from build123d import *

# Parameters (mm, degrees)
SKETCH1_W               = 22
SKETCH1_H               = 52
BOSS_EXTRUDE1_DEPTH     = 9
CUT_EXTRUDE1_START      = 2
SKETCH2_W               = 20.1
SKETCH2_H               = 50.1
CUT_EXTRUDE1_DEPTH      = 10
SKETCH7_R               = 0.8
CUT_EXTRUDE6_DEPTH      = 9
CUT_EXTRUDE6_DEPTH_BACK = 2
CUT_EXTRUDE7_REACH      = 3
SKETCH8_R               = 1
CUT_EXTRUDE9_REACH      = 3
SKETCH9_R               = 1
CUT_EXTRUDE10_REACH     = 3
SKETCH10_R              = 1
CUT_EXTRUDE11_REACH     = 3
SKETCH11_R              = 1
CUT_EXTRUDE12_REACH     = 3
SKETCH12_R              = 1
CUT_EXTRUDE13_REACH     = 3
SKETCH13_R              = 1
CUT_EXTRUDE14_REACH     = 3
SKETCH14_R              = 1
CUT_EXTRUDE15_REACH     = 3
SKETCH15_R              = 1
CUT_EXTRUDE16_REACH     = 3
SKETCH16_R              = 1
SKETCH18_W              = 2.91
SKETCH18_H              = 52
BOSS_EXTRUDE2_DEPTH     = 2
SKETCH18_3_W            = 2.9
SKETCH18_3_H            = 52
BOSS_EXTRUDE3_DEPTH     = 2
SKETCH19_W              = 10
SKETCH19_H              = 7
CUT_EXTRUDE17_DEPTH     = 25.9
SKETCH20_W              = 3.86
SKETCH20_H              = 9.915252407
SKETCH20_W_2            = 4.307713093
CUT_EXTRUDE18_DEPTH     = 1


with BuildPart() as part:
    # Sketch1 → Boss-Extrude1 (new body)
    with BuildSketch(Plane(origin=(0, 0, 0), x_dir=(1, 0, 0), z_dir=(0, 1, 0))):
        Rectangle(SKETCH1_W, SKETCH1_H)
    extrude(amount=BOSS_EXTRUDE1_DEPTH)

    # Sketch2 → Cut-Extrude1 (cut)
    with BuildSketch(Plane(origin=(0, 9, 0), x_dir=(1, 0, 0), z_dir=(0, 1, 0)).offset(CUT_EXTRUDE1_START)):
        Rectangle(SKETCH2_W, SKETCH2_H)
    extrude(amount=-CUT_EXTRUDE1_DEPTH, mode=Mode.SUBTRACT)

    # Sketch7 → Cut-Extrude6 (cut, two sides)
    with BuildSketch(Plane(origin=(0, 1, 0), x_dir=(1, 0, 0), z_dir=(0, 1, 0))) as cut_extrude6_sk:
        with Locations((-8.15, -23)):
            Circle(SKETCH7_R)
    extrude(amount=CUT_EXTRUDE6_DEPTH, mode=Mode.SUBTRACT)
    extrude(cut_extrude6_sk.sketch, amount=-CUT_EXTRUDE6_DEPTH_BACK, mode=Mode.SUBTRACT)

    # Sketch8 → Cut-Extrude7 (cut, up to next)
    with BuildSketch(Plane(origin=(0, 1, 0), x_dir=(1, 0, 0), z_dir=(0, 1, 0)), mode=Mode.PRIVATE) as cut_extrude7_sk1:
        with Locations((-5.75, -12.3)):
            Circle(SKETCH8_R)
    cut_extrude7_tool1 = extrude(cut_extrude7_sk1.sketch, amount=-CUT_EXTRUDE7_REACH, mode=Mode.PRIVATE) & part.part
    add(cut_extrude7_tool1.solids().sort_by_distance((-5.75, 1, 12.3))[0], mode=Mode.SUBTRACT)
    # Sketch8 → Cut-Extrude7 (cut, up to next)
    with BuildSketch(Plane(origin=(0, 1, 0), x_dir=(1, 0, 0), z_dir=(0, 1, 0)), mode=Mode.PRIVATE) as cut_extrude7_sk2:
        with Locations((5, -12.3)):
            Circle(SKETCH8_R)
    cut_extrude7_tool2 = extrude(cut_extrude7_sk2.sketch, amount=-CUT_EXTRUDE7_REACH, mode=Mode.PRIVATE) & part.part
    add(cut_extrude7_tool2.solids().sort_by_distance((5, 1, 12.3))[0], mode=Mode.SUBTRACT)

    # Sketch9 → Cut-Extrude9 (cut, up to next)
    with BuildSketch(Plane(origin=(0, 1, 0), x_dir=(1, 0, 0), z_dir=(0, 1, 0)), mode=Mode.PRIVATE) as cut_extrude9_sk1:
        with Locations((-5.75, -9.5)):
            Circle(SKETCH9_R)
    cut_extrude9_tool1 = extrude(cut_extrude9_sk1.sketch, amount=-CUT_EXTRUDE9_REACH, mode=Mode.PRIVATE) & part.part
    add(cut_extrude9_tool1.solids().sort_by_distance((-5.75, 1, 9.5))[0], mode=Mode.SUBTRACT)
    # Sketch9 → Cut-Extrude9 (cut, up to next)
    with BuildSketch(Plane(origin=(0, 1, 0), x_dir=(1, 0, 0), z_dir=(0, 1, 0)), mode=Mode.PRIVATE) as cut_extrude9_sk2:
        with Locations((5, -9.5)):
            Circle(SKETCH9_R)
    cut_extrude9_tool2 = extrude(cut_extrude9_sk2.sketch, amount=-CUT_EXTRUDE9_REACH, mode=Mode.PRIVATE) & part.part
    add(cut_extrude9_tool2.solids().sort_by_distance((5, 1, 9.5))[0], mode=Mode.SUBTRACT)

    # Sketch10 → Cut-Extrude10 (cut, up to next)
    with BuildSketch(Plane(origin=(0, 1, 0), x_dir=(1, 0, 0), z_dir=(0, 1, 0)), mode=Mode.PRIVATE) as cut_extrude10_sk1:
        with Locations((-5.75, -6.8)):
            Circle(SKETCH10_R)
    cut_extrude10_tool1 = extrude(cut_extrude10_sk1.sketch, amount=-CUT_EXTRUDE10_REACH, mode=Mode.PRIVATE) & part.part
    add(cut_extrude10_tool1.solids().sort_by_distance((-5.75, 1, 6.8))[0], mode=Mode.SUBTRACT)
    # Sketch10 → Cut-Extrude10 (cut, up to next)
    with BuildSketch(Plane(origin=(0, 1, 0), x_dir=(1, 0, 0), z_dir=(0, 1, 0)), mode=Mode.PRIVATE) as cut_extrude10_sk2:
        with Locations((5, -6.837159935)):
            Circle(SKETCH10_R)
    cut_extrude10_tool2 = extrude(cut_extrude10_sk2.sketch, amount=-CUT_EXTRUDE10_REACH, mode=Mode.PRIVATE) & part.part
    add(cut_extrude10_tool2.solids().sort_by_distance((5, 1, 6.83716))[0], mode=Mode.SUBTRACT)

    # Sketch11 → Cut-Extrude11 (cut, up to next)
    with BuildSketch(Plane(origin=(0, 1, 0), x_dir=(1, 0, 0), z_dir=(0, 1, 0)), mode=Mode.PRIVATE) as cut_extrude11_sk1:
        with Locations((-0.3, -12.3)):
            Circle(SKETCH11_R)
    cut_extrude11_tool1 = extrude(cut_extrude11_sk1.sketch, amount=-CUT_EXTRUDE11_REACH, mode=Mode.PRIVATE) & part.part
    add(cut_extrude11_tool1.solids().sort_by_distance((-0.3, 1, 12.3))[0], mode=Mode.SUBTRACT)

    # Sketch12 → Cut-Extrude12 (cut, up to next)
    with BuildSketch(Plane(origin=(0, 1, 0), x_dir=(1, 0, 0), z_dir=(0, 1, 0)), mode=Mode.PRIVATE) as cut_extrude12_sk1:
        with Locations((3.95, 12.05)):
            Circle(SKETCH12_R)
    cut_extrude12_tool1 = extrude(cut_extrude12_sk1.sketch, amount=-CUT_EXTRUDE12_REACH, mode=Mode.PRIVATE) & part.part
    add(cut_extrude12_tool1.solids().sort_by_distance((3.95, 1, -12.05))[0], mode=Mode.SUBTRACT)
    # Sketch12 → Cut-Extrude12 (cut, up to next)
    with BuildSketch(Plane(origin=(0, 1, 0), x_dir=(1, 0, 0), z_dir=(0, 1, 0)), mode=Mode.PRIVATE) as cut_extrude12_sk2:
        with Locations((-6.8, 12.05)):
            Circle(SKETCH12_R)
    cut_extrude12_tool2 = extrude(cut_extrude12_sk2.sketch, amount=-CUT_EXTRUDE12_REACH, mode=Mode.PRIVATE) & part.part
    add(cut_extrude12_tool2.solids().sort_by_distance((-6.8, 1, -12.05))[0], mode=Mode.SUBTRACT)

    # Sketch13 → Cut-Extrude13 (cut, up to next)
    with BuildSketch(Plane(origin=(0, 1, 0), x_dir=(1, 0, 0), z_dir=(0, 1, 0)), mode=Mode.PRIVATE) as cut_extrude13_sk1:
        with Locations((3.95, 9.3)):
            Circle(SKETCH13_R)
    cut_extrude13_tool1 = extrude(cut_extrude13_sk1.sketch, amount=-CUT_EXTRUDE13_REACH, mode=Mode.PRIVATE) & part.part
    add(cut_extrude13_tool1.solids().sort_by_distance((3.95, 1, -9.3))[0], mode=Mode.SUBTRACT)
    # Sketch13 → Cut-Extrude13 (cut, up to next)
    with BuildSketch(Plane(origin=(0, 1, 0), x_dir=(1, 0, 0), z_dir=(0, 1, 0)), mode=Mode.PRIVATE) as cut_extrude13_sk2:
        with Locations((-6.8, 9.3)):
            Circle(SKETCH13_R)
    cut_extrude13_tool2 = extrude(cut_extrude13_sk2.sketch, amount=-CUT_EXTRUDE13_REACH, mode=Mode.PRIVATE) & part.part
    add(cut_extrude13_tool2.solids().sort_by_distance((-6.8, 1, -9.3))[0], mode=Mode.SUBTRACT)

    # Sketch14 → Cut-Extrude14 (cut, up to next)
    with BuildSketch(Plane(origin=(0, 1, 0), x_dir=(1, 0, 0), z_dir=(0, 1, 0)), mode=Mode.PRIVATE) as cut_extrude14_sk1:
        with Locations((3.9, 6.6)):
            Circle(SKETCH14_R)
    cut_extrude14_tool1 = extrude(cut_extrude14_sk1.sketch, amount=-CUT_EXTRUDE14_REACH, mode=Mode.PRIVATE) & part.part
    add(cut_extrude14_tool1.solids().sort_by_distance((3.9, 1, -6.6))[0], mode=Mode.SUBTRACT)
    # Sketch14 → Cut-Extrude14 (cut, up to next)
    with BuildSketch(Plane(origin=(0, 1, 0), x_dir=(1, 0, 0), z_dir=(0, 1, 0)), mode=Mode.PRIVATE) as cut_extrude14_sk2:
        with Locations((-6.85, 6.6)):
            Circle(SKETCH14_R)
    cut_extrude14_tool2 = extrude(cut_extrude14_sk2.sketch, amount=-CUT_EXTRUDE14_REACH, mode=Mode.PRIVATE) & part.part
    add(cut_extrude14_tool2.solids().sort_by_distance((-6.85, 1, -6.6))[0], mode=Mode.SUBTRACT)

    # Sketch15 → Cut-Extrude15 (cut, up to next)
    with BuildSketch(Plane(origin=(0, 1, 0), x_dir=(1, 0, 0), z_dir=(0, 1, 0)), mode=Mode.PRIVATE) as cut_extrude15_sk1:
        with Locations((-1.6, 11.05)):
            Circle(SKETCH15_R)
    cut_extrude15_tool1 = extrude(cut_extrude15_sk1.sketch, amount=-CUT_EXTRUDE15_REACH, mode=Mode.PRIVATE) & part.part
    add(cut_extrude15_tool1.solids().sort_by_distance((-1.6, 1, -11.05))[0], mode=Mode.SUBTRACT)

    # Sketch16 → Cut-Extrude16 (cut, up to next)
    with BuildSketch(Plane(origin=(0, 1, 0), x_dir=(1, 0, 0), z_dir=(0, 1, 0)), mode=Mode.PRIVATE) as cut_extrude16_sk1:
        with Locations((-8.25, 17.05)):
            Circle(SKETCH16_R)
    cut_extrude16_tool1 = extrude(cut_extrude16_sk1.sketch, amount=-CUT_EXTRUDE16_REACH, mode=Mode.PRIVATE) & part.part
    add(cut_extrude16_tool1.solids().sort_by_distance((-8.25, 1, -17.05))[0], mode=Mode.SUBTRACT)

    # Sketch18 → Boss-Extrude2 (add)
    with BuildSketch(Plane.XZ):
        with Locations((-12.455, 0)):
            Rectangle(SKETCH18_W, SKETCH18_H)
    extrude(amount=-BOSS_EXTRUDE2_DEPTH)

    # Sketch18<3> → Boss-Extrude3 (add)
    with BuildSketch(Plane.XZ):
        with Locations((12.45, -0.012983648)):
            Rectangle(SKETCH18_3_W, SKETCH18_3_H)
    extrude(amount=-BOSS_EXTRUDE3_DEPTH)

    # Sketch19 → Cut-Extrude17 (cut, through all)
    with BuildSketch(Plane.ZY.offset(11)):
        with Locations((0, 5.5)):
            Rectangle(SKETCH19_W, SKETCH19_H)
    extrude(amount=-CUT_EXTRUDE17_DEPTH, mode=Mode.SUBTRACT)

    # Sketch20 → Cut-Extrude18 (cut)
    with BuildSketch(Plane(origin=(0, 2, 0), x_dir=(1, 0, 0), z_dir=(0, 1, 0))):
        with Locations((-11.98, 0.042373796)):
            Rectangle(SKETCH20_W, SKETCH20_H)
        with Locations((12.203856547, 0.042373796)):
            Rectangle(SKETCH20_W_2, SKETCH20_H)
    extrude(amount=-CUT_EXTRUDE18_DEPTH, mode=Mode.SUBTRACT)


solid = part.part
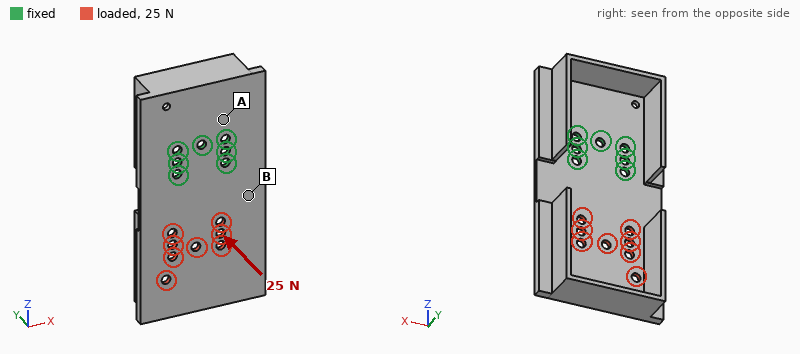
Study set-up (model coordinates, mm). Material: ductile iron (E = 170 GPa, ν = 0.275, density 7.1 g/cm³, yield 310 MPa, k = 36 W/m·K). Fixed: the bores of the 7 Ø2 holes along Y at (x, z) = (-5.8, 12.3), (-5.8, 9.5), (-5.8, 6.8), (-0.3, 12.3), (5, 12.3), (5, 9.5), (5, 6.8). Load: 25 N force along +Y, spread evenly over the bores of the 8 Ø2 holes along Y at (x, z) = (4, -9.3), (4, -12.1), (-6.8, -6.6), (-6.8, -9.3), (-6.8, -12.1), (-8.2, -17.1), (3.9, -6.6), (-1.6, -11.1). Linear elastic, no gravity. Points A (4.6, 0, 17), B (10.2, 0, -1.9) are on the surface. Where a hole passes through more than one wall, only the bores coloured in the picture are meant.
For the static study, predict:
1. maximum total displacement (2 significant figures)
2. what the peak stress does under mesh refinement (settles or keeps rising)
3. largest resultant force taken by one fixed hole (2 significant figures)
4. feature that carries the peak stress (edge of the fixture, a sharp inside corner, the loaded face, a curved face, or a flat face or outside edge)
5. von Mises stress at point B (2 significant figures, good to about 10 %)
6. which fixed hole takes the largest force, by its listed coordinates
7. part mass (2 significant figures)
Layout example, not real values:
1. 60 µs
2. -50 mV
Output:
1. 0.24 mm
2. keeps rising
3. 34 N
4. edge of the fixture
5. 46 MPa
6. (-5.8, 6.8)
7. 18 g
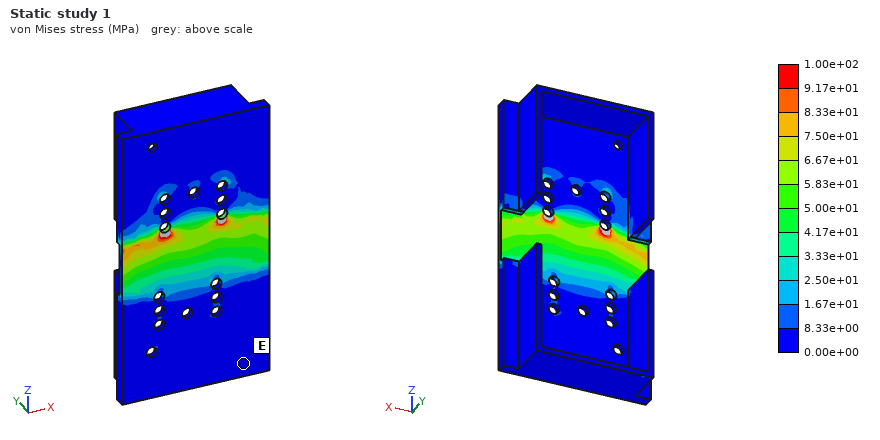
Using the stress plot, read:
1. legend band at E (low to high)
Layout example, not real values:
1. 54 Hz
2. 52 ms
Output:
1. 0.00e+00 to 8.33e+00 MPa
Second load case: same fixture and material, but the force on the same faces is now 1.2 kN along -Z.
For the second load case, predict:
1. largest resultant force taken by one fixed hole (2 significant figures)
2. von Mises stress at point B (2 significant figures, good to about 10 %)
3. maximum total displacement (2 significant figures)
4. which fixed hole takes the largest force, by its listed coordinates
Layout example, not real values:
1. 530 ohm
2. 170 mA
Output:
1. 450 N
2. 22 MPa
3. 13 µm
4. (-5.8, 6.8)
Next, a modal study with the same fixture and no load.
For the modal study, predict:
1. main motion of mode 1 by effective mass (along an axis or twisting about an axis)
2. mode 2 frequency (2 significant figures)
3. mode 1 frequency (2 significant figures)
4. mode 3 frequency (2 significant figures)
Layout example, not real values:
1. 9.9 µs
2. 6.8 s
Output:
1. along Y
2. 1600 Hz
3. 530 Hz
4. 3900 Hz
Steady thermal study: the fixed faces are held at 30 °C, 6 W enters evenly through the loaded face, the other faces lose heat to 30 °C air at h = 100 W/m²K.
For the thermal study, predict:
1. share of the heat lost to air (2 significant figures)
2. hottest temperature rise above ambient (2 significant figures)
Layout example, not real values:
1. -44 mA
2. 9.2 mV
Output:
1. 79 %
2. 40 K
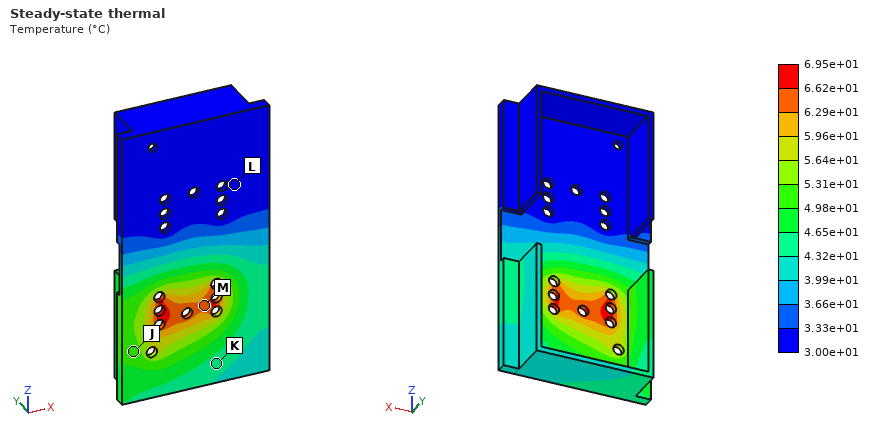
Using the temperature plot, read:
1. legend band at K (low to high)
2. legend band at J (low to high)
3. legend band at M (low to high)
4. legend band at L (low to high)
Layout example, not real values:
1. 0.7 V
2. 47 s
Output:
1. 4.32e+01 to 4.65e+01 °C
2. 4.98e+01 to 5.31e+01 °C
3. 6.29e+01 to 6.62e+01 °C
4. 3.00e+01 to 3.33e+01 °C
